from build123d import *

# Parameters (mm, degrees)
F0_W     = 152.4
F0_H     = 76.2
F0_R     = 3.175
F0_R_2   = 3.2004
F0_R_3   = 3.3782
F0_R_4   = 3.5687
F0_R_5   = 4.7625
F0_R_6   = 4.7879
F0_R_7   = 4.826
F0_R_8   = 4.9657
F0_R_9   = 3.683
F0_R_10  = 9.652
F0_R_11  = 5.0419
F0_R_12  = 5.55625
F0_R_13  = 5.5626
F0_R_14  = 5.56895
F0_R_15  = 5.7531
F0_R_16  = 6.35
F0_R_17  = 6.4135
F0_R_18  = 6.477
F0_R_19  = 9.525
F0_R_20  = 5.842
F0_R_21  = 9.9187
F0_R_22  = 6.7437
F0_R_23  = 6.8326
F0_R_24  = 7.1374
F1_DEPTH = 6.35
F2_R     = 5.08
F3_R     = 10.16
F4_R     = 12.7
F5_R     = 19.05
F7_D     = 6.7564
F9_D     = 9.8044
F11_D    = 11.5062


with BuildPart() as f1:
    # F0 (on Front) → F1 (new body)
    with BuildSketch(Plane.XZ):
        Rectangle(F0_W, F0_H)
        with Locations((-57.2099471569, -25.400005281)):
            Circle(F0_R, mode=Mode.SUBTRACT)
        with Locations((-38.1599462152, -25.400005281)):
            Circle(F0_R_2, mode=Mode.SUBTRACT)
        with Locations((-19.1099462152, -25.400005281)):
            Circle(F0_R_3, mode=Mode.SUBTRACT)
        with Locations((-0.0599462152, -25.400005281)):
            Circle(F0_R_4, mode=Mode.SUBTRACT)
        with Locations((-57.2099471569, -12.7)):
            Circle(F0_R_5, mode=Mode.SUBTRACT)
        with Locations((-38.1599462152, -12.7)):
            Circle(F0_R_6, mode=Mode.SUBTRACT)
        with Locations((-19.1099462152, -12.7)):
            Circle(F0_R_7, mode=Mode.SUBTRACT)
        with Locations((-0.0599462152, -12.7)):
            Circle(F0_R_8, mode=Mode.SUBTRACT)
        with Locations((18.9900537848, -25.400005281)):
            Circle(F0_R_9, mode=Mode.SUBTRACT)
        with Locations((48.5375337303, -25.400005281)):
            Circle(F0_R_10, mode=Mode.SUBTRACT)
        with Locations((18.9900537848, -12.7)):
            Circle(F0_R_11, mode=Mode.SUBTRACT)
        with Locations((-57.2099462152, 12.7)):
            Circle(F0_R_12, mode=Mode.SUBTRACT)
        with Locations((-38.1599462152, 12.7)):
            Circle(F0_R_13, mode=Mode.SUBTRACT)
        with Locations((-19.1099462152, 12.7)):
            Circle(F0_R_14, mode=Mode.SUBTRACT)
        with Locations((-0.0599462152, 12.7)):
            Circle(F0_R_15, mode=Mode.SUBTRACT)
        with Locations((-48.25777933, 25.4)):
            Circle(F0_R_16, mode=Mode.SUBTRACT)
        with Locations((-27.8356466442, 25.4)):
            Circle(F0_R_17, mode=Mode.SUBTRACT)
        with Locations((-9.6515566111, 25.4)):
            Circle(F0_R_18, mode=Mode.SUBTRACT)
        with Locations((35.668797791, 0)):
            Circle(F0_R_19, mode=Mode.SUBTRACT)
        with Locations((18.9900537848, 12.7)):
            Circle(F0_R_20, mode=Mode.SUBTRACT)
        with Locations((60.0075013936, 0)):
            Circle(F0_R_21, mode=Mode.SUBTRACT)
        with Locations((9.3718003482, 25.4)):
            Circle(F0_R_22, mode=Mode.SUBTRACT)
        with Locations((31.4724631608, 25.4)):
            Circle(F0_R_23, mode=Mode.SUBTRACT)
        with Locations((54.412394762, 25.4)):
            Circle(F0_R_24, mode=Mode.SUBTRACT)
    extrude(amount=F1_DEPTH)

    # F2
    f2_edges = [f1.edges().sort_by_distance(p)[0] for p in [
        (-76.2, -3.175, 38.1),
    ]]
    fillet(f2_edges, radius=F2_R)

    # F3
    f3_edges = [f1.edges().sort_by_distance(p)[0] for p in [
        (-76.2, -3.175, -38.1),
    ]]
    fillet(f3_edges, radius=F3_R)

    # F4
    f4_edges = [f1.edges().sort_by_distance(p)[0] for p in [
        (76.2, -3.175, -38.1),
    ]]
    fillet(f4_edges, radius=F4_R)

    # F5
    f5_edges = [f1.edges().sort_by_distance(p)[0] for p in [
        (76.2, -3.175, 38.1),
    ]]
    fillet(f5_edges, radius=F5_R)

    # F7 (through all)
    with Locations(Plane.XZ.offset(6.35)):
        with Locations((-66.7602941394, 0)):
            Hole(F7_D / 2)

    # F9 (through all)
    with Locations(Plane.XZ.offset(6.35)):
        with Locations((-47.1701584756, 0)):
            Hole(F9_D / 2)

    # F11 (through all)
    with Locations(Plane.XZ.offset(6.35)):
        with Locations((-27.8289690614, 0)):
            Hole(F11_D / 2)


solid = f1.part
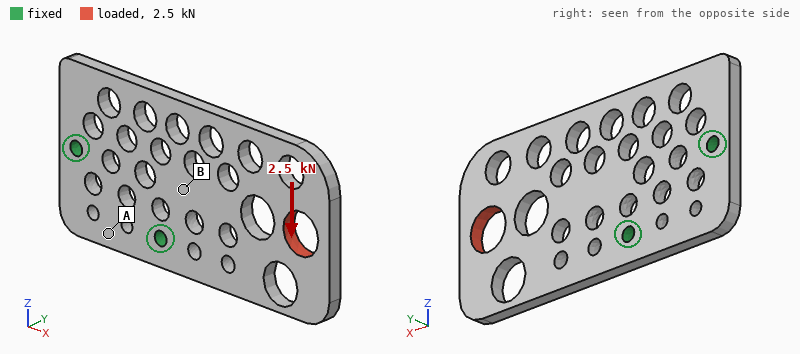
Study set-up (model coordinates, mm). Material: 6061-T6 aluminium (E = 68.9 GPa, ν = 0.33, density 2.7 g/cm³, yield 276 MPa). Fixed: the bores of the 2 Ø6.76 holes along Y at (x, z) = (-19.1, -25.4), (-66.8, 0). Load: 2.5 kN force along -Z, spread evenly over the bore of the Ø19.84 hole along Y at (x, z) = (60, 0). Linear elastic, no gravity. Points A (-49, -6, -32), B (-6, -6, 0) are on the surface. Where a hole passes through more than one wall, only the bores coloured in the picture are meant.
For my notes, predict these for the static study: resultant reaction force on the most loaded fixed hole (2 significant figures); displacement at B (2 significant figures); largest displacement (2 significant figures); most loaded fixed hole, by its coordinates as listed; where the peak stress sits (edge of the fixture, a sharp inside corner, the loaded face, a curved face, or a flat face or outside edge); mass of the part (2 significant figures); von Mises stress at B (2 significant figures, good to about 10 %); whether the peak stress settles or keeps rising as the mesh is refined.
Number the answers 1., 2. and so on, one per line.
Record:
1. 5.3 kN
2. 0.037 mm
3. 0.22 mm
4. (-19.1, -25.4)
5. edge of the fixture
6. 150 g
7. 22 MPa
8. keeps rising
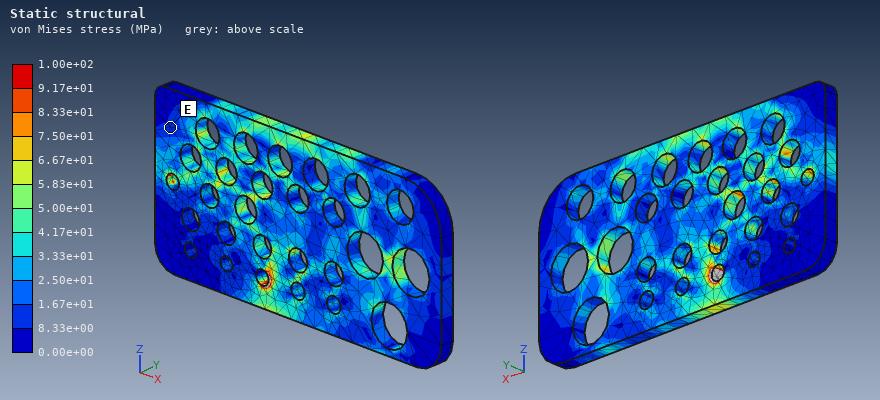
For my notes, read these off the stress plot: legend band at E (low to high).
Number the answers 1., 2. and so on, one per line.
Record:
1. 8.33e+00 to 1.67e+01 MPa
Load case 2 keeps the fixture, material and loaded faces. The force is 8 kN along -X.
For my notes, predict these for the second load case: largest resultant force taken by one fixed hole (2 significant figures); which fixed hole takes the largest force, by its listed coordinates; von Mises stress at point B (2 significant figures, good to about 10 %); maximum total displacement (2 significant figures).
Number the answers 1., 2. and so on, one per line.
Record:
1. 5.2 kN
2. (-19.1, -25.4)
3. 28 MPa
4. 0.15 mm
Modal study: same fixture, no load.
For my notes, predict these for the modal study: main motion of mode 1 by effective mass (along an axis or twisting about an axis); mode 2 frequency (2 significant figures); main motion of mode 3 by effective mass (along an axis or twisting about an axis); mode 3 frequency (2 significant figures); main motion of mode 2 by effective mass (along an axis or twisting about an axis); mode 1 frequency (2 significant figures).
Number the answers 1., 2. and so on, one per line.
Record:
1. along Y
2. 1100 Hz
3. along Y
4. 2100 Hz
5. twisting about X
6. 450 Hz
